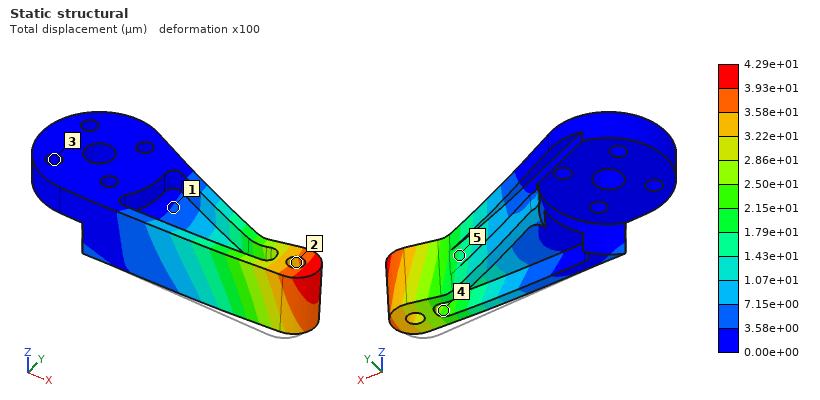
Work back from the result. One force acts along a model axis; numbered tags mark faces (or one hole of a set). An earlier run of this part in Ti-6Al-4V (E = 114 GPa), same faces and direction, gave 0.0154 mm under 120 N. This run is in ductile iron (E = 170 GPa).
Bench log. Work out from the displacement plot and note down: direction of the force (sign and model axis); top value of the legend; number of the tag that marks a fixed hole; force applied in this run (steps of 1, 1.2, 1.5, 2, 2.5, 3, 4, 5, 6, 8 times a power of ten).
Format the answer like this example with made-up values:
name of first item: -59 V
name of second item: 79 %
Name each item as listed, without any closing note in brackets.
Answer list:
direction of the force: +Y
top value of the legend: 4.29e+01 µm
number of the tag that marks a fixed hole: 3
force applied in this run: 500 N
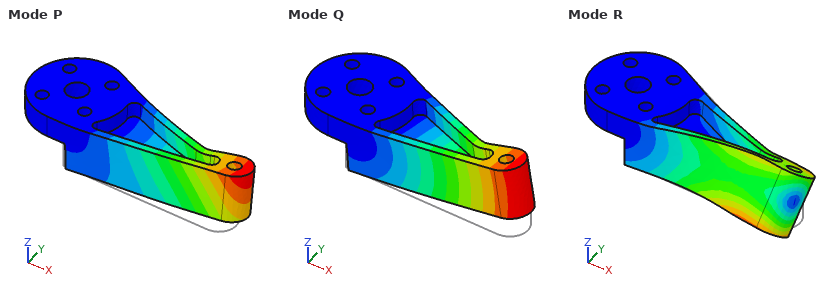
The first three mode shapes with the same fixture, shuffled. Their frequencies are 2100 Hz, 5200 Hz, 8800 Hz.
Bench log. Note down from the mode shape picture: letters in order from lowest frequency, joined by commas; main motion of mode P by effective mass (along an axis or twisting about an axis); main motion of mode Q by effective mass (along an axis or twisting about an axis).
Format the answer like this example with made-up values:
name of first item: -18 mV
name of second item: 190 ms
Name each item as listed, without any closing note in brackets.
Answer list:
letters in order from lowest frequency, joined by commas: Q, P, R
main motion of mode P by effective mass: along Y
main motion of mode Q by effective mass: along Z
